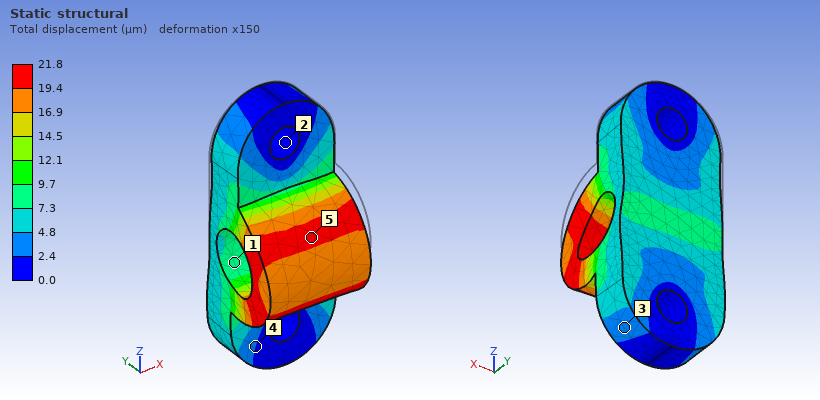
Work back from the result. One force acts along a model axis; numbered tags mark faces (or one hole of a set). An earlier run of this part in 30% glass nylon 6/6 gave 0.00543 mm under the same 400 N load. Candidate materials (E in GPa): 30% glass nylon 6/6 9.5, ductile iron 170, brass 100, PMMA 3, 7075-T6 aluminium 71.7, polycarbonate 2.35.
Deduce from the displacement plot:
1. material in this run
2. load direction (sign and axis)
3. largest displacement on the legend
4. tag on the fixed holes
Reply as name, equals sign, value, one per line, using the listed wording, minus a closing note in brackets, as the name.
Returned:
material in this run = polycarbonate
load direction = -Z
largest displacement on the legend = 21.8 µm
tag on the fixed holes = 2
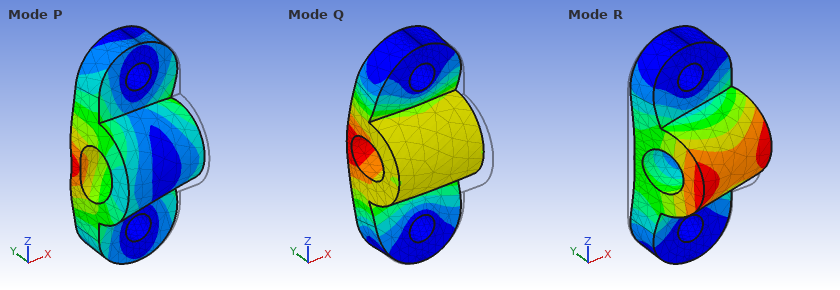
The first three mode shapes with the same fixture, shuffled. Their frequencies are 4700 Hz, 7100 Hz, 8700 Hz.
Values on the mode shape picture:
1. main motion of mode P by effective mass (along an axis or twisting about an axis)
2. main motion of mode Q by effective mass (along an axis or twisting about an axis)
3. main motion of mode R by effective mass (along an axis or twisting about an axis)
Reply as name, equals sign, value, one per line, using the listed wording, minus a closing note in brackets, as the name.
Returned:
main motion of mode P by effective mass = along X
main motion of mode Q by effective mass = along Y
main motion of mode R by effective mass = along X
